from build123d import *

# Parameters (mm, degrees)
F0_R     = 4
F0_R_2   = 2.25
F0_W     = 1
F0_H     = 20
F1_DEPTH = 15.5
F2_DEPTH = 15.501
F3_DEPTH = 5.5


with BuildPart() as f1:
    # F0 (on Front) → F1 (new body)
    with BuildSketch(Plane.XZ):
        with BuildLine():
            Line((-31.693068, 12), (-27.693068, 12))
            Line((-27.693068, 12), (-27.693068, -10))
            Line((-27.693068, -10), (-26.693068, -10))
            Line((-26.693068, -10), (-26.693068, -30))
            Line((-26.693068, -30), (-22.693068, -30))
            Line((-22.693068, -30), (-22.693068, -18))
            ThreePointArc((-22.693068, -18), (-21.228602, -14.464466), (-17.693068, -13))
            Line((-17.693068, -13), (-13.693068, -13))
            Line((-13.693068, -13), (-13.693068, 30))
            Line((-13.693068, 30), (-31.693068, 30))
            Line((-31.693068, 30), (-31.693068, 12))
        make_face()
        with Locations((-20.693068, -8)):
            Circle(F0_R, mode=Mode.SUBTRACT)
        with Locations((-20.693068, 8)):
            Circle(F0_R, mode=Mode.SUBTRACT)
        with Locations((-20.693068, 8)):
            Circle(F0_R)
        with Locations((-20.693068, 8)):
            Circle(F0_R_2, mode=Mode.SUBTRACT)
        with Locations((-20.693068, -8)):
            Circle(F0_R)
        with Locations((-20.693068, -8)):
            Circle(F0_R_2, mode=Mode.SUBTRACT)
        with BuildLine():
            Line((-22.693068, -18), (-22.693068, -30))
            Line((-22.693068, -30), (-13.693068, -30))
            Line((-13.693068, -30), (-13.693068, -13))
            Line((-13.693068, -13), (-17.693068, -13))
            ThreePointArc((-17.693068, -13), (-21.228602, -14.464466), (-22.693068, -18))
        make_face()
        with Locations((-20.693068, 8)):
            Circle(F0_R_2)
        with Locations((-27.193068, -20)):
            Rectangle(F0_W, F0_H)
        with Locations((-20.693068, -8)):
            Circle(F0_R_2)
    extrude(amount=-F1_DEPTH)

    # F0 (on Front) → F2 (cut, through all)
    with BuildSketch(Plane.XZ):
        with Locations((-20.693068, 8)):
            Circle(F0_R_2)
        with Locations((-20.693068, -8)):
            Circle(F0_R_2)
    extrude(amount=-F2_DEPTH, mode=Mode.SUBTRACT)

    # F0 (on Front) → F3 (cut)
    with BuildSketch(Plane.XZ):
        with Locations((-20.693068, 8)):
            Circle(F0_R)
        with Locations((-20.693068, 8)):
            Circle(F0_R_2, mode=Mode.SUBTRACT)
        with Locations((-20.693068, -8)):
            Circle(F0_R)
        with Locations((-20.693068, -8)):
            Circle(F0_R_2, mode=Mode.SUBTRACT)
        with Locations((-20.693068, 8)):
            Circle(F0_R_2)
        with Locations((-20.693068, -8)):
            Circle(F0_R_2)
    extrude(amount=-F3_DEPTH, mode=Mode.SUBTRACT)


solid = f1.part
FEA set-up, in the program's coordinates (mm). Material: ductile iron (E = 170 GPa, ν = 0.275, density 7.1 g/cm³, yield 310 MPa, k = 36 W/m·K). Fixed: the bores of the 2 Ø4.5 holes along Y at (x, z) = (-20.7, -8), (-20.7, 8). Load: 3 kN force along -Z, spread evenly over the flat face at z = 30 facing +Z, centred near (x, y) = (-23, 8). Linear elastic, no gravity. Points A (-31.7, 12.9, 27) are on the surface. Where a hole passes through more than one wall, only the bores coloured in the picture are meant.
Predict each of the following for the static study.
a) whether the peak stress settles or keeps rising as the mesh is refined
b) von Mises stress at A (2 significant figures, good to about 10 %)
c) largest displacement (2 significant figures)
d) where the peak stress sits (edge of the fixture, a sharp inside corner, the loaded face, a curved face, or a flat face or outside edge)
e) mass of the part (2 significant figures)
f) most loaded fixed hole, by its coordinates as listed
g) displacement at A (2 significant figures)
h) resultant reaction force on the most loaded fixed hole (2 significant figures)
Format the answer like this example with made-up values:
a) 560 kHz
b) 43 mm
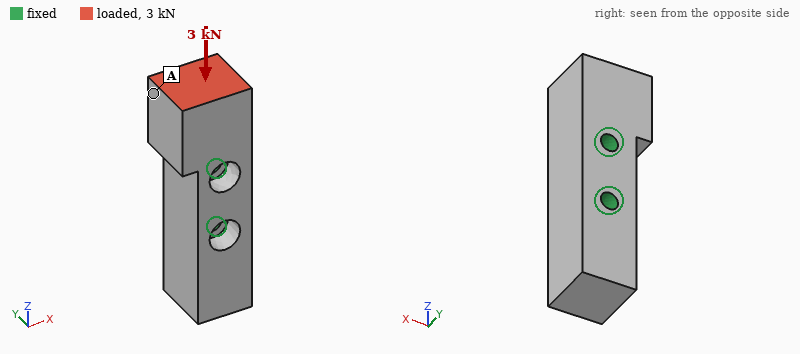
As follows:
a) keeps rising
b) 11 MPa
c) 5.5 µm
d) edge of the fixture
e) 94 g
f) (-20.7, 8)
g) 4.0 µm
h) 2.5 kN
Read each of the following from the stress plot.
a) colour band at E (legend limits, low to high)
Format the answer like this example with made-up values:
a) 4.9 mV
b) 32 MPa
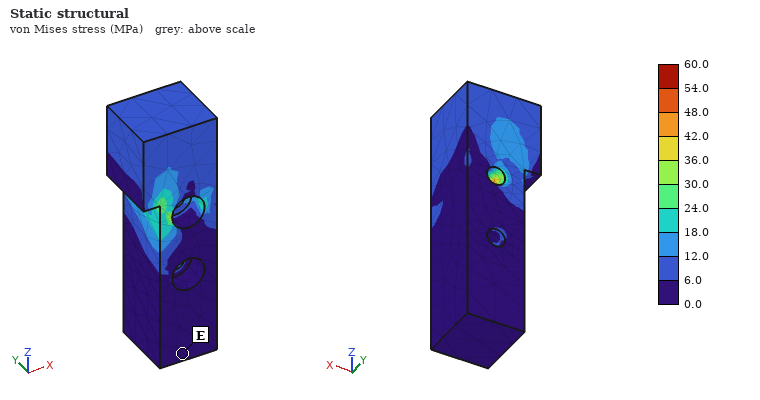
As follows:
a) 0.0 to 6.0 MPa
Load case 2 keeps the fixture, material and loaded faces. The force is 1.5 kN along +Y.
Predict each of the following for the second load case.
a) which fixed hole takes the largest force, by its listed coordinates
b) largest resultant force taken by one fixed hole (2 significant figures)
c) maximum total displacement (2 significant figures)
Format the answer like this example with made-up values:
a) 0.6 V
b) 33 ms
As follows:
a) (-20.7, 8)
b) 2.3 kN
c) 17 µm
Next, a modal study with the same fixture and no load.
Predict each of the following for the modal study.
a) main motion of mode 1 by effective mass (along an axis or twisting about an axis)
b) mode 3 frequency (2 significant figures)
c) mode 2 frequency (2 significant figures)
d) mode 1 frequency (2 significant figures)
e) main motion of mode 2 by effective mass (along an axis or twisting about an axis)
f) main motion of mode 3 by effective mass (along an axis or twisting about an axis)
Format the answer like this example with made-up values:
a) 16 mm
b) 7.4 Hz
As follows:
a) along X
b) 14 kHz
c) 13 kHz
d) 12 kHz
e) along Y
f) along X
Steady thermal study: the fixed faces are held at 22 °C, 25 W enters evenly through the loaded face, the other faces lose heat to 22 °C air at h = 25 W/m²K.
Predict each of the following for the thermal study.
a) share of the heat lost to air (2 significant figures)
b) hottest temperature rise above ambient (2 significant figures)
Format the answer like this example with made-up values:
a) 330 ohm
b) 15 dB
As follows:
a) 5.9 %
b) 63 K
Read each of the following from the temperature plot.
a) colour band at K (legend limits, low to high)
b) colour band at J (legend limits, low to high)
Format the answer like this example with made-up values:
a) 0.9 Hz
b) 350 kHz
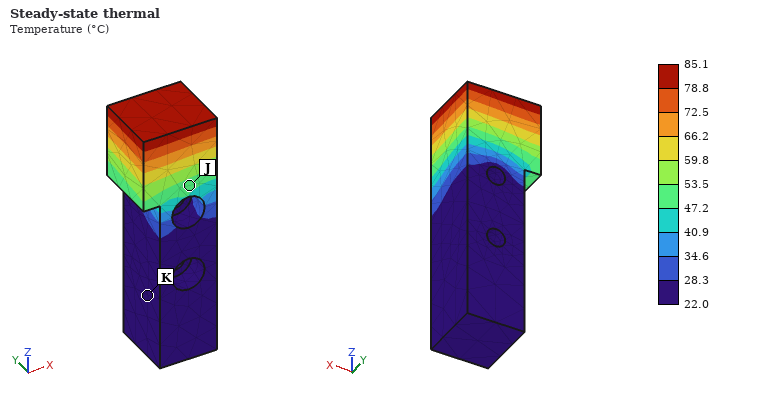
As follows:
a) 22.0 to 28.3 °C
b) 47.2 to 53.5 °C
